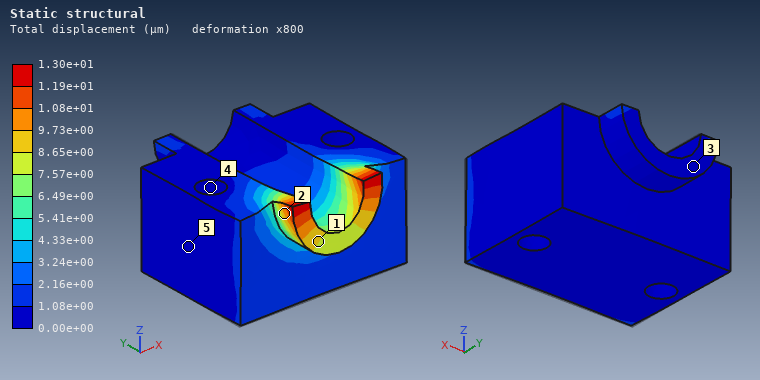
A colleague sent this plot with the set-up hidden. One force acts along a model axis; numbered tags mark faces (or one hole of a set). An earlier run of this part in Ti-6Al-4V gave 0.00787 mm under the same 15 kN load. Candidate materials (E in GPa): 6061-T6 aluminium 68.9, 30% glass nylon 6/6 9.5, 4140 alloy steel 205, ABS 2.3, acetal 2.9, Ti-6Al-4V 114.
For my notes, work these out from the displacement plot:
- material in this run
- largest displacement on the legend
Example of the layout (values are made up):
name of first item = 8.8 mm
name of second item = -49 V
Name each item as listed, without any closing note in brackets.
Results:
material in this run = 6061-T6 aluminium
largest displacement on the legend = 1.30e+01 µm
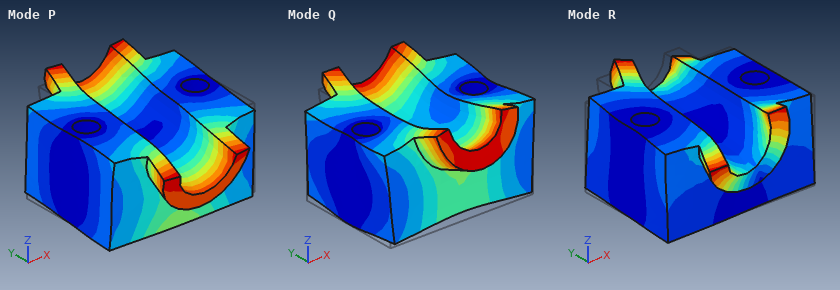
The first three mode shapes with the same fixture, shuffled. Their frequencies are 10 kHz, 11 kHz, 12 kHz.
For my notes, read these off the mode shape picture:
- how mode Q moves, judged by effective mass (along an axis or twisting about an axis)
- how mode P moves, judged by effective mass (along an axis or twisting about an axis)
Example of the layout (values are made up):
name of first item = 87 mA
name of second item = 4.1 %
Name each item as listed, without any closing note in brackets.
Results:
how mode Q moves, judged by effective mass = along Z
how mode P moves, judged by effective mass = twisting about X
